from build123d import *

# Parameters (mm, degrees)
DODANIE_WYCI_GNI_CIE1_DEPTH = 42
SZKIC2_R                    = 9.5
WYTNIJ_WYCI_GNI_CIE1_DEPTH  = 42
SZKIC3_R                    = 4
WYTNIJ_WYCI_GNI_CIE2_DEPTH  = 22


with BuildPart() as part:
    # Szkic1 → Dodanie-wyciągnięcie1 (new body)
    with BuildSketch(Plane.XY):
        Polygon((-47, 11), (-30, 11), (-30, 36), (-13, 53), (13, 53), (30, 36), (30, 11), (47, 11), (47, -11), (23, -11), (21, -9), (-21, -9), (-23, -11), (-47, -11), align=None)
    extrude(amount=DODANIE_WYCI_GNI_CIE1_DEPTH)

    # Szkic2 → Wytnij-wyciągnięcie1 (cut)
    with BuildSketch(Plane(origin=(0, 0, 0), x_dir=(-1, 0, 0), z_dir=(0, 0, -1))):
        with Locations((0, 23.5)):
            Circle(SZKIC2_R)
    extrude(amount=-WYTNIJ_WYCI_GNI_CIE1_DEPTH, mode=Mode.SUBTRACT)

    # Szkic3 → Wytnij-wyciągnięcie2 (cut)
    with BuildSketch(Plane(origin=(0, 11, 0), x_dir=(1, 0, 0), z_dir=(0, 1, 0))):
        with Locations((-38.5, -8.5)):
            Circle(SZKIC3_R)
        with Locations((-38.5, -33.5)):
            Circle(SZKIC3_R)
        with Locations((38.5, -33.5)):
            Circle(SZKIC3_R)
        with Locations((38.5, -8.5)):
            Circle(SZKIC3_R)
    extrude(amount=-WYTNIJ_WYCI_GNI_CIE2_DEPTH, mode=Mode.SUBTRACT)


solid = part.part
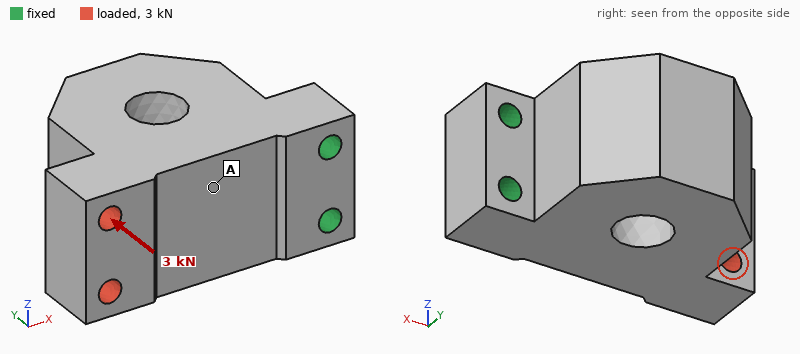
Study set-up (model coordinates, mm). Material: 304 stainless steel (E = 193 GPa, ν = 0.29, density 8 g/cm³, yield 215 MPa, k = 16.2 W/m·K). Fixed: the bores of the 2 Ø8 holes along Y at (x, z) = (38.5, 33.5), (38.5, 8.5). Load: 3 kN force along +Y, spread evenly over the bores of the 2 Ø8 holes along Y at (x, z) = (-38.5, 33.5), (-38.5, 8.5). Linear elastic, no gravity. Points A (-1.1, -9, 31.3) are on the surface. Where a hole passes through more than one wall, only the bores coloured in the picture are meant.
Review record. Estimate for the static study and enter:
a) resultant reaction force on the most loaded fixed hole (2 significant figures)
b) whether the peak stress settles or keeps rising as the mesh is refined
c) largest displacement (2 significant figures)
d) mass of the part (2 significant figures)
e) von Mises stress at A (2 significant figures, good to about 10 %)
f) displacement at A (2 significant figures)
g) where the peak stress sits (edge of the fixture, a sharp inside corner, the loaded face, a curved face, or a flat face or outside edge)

1.5 kN
keeps rising
53 µm
1.3 kg
13 MPa
20 µm
edge of the fixture
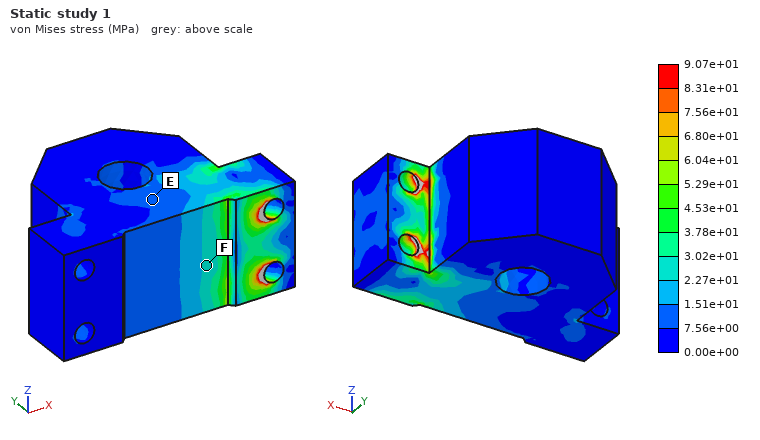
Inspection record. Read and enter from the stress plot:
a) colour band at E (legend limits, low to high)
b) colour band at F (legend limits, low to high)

7.56e+00 to 1.51e+01 MPa
2.27e+01 to 3.02e+01 MPa
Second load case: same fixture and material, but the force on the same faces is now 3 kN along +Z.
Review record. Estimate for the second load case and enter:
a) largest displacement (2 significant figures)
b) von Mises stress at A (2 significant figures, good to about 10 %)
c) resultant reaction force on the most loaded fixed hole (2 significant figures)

24 µm
11 MPa
7.9 kN
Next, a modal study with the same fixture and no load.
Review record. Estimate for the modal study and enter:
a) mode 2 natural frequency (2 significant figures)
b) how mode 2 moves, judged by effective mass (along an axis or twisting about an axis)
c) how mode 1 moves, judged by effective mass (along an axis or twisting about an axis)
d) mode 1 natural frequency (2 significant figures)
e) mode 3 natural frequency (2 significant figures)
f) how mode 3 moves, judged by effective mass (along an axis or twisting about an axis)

3200 Hz
along Z
along Y
1800 Hz
4600 Hz
twisting about X
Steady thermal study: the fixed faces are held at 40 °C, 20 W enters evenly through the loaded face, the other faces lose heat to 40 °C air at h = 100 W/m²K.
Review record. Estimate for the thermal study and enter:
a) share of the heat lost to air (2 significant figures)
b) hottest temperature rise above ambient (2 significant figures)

87 %
32 K
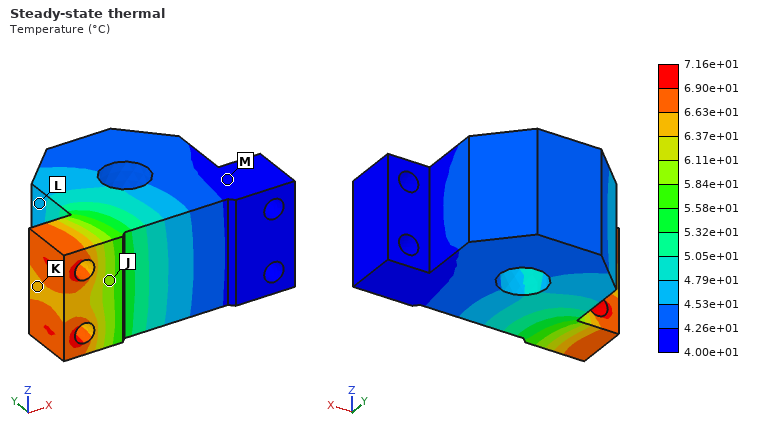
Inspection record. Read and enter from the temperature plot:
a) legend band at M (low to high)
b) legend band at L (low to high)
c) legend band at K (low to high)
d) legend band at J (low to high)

4.00e+01 to 4.26e+01 °C
4.53e+01 to 4.79e+01 °C
6.37e+01 to 6.63e+01 °C
5.84e+01 to 6.11e+01 °C
